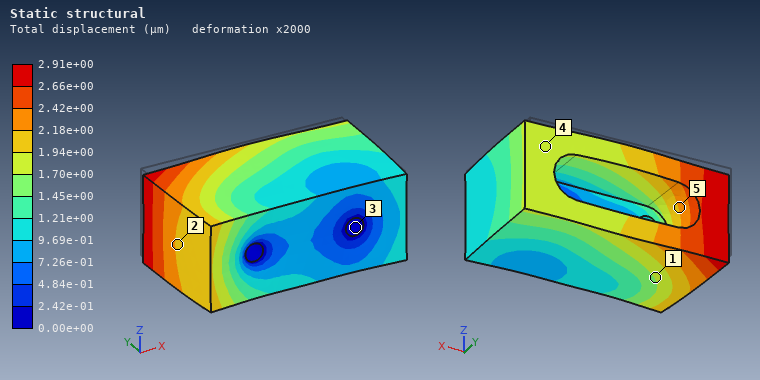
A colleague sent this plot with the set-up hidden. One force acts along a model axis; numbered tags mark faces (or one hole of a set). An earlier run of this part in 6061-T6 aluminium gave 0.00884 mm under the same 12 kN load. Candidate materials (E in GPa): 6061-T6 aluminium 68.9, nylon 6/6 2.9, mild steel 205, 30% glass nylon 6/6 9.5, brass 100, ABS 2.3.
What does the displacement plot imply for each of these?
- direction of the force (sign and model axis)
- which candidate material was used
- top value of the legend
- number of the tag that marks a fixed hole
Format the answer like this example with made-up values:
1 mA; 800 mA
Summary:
-Y; mild steel; 2.91e+00 µm; 3
